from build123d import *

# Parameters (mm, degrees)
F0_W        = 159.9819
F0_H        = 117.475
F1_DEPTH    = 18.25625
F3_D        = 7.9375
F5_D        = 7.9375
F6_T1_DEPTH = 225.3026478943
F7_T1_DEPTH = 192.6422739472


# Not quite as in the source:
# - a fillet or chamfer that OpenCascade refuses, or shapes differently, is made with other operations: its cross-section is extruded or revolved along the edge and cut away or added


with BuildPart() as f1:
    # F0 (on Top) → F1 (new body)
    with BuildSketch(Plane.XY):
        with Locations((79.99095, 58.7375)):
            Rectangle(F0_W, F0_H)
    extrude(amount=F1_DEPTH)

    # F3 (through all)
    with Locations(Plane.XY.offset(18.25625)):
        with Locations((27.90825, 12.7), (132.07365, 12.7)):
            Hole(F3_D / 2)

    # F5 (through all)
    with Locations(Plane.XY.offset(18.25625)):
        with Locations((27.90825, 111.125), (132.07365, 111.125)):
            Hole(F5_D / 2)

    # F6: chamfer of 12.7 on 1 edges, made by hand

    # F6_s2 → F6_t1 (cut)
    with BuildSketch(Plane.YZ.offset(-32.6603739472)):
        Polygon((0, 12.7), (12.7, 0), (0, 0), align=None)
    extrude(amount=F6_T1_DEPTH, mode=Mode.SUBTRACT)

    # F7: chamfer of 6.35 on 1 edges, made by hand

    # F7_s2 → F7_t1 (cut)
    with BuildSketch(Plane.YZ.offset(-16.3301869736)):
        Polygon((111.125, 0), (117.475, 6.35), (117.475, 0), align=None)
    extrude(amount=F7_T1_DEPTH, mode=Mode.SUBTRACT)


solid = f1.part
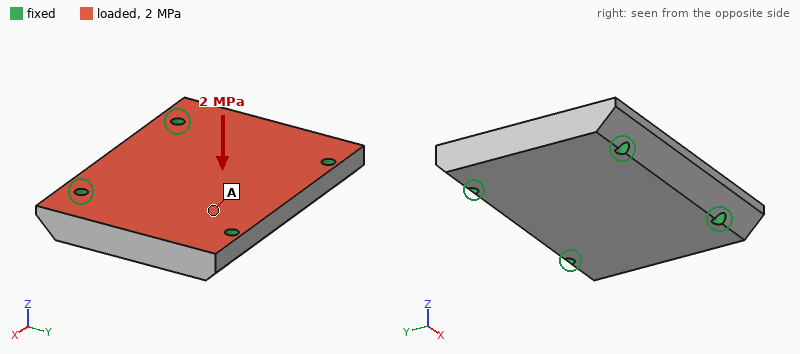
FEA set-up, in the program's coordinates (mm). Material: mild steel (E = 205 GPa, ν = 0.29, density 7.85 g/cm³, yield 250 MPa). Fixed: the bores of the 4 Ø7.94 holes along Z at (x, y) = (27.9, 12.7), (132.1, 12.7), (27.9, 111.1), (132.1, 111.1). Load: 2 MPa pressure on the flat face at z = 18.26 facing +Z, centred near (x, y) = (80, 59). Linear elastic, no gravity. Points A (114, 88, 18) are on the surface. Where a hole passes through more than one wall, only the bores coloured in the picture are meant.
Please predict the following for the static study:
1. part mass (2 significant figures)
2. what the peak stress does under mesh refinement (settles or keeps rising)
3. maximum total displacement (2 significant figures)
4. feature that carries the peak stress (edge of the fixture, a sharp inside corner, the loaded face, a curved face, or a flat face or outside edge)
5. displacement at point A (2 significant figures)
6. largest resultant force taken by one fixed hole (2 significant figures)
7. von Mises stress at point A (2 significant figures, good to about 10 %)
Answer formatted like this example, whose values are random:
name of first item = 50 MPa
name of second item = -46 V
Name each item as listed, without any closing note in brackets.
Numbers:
part mass = 2.5 kg
what the peak stress does under mesh refinement = keeps rising
maximum total displacement = 19 µm
feature that carries the peak stress = edge of the fixture
displacement at point A = 12 µm
largest resultant force taken by one fixed hole = 9.9 kN
von Mises stress at point A = 10.0 MPa
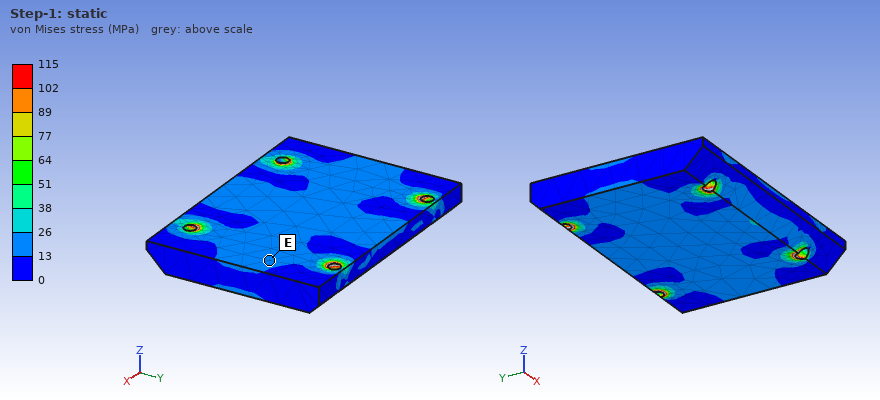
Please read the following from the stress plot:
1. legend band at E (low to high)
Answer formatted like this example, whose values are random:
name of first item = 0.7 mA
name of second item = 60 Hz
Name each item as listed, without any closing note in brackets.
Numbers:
legend band at E = 13 to 26 MPa
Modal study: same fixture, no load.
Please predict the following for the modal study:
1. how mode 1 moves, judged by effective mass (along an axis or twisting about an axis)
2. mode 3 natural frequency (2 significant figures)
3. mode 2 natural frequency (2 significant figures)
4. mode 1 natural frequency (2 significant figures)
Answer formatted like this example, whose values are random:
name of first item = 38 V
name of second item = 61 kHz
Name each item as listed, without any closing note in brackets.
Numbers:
how mode 1 moves, judged by effective mass = along Z
mode 3 natural frequency = 7100 Hz
mode 2 natural frequency = 6900 Hz
mode 1 natural frequency = 5100 Hz
